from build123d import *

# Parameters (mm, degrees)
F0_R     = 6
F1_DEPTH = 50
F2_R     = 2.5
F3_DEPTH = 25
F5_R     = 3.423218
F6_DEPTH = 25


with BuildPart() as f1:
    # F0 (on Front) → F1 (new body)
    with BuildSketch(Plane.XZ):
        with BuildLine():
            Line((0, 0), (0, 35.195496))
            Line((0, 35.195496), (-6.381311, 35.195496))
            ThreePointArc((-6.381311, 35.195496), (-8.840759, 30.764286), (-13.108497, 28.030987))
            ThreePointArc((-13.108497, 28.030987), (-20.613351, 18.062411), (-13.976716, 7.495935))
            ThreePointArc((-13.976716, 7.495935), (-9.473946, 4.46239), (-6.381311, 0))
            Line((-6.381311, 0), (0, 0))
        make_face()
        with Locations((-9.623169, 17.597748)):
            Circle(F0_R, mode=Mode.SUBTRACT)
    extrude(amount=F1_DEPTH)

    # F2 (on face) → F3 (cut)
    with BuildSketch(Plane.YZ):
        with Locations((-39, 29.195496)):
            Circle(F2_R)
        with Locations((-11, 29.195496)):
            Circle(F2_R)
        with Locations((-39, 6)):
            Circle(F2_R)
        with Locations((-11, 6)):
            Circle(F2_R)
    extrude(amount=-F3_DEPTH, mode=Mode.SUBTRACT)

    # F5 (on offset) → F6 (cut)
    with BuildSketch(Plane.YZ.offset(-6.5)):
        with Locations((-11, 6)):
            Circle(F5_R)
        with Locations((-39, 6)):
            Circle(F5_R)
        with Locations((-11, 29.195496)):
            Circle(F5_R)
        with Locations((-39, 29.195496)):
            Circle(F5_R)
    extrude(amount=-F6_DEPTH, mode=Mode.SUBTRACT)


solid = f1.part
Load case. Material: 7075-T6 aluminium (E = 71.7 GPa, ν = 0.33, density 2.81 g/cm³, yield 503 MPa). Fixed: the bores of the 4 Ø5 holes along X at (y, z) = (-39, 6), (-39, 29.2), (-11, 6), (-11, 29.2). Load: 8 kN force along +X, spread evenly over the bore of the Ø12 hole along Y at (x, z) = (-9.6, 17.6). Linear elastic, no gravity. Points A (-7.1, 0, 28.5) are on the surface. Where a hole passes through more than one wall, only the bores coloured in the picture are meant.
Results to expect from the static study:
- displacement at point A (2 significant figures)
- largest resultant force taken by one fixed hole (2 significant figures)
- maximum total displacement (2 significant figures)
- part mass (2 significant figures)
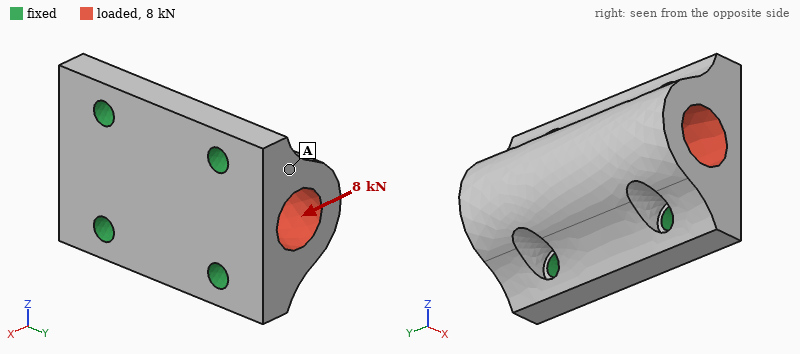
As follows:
3.8 µm
2.0 kN
6.9 µm
53 g
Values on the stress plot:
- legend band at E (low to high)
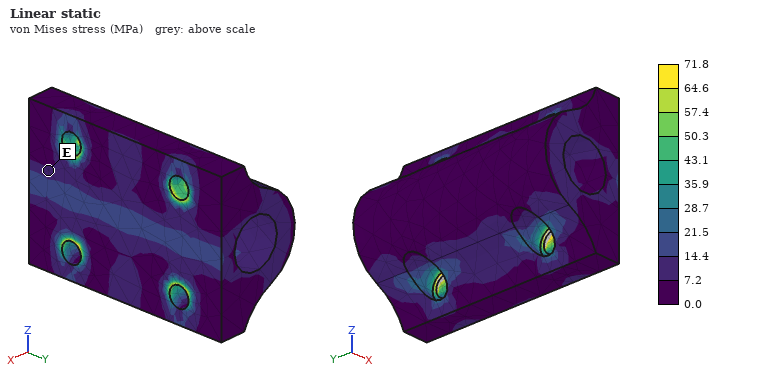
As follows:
7.2 to 14.4 MPa
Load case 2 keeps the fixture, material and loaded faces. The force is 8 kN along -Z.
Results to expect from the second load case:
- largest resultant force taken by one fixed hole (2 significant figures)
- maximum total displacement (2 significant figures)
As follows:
2.2 kN
9.5 µm
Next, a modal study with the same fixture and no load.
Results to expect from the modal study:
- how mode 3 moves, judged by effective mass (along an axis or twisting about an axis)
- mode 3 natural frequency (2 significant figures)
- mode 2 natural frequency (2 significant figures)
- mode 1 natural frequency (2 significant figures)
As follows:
twisting about X
32 kHz
26 kHz
26 kHz
